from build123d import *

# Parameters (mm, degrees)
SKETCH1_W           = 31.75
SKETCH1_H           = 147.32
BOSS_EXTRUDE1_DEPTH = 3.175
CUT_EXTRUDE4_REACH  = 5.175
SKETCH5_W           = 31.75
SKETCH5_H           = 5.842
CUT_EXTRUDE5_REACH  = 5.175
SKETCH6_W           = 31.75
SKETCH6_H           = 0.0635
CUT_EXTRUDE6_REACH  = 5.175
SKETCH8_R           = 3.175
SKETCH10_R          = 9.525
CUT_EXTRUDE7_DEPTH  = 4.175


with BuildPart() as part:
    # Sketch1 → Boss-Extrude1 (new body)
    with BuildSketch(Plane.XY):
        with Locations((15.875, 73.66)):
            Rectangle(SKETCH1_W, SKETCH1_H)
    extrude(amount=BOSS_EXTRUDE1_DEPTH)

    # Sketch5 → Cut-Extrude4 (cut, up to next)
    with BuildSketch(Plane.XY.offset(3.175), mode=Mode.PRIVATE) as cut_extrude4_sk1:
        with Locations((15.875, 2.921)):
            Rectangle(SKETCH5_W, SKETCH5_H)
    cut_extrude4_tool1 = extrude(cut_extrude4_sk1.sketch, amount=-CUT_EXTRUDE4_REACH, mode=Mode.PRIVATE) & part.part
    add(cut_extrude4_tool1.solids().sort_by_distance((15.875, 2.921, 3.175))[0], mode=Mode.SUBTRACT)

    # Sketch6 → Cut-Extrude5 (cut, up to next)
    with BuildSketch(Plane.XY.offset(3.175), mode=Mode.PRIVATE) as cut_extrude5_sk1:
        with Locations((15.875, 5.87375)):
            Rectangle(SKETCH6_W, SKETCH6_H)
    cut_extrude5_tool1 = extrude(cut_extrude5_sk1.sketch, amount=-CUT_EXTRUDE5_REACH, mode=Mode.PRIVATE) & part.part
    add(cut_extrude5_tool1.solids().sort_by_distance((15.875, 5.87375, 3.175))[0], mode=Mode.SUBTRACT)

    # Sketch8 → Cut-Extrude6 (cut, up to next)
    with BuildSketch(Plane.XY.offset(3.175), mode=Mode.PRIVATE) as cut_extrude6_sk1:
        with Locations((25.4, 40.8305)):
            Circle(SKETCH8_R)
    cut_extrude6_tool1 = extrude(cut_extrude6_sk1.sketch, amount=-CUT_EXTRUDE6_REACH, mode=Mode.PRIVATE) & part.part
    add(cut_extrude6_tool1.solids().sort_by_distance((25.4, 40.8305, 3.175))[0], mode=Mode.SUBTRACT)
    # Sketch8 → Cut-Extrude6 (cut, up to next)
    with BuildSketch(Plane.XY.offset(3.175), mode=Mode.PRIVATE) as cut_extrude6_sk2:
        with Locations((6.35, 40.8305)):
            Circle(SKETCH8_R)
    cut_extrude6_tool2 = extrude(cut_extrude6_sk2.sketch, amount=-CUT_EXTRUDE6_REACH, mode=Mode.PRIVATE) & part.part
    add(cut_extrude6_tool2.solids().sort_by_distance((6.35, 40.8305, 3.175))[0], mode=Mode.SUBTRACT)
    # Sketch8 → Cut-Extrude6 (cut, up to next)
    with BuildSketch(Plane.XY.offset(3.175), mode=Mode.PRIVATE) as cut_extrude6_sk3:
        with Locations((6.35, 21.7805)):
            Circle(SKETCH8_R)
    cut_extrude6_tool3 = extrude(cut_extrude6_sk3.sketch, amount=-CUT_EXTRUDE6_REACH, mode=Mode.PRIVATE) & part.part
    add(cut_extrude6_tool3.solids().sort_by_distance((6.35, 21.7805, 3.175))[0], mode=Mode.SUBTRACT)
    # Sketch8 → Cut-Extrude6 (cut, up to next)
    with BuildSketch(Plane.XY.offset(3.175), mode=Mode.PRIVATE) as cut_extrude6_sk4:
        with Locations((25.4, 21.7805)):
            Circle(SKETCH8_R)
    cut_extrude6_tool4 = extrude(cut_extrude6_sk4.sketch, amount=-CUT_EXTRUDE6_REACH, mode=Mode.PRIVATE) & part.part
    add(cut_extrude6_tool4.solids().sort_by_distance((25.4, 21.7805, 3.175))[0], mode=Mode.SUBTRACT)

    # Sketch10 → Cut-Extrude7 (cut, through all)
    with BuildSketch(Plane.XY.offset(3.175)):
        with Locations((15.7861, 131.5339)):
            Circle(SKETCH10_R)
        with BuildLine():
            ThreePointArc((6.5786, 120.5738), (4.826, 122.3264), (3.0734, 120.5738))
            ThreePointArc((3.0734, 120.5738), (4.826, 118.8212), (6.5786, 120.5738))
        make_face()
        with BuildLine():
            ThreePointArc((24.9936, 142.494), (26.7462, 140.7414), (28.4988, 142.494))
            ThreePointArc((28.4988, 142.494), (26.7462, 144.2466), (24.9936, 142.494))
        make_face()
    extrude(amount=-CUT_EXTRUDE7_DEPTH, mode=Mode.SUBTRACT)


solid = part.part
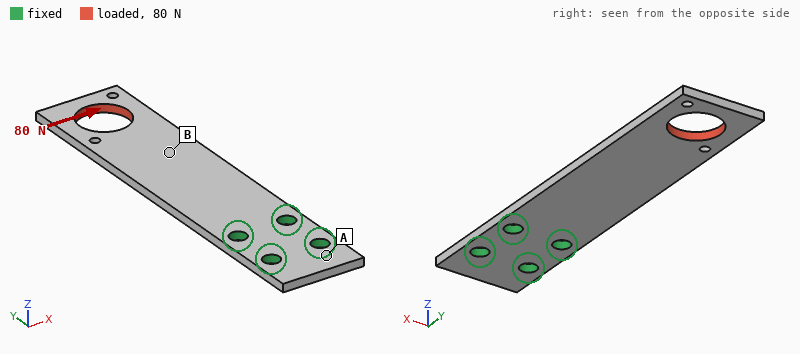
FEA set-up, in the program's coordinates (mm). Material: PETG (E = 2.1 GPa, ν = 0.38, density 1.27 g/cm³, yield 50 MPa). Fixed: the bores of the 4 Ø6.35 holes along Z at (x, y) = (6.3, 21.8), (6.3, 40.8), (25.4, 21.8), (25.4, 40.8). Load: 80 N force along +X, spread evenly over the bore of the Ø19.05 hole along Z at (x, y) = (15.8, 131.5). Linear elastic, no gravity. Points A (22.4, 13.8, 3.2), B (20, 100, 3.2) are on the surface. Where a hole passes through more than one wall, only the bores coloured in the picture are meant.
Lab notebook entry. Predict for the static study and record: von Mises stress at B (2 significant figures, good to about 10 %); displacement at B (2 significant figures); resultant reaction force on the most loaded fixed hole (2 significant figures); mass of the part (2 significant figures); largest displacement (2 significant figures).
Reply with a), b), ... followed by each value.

a) 2.3 MPa
b) 0.61 mm
c) 310 N
d) 16 g
e) 1.6 mm
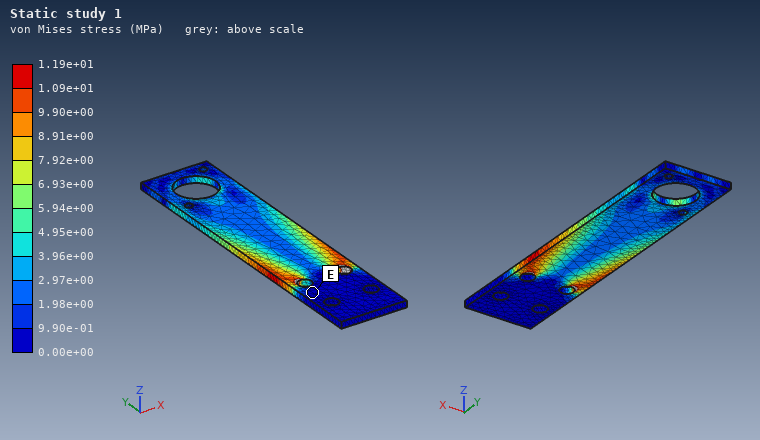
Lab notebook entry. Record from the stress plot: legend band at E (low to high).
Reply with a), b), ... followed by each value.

a) 0.00e+00 to 9.90e-01 MPa
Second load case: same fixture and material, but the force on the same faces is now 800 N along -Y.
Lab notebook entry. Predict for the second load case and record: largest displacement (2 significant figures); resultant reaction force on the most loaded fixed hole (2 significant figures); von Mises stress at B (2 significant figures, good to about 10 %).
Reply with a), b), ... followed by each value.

a) 0.58 mm
b) 380 N
c) 7.2 MPa
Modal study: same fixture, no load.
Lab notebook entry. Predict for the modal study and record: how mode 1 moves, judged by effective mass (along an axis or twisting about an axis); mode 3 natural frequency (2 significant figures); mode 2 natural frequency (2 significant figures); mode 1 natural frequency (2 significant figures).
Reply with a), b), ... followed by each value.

a) along Z
b) 390 Hz
c) 380 Hz
d) 70 Hz
